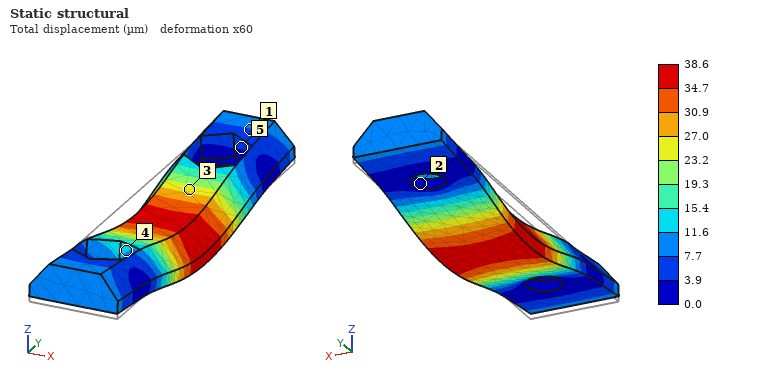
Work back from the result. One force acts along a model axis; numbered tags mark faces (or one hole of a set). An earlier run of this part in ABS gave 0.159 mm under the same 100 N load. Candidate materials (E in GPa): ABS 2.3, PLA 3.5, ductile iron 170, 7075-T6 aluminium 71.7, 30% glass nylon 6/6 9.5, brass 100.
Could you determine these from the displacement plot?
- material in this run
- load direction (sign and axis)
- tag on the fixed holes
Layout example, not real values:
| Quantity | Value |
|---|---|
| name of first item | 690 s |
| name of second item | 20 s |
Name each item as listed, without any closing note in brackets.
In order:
| Quantity | Value |
|---|---|
| material in this run | 30% glass nylon 6/6 |
| load direction | -Z |
| tag on the fixed holes | 2 |
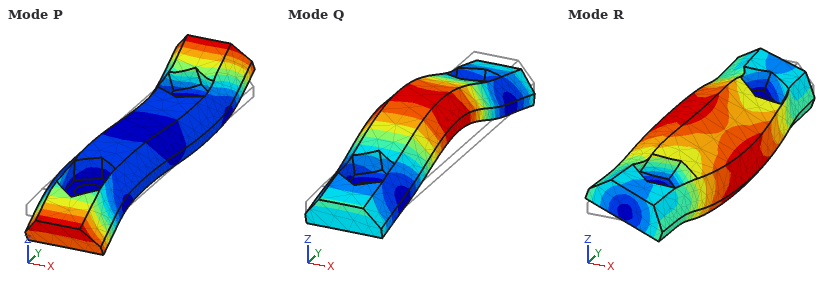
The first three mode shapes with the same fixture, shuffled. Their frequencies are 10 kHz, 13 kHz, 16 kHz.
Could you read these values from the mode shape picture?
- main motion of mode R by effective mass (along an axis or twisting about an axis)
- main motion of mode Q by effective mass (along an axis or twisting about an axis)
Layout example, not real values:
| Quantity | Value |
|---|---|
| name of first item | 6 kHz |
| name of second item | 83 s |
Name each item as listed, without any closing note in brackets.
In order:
| Quantity | Value |
|---|---|
| main motion of mode R by effective mass | along X |
| main motion of mode Q by effective mass | along Z |
